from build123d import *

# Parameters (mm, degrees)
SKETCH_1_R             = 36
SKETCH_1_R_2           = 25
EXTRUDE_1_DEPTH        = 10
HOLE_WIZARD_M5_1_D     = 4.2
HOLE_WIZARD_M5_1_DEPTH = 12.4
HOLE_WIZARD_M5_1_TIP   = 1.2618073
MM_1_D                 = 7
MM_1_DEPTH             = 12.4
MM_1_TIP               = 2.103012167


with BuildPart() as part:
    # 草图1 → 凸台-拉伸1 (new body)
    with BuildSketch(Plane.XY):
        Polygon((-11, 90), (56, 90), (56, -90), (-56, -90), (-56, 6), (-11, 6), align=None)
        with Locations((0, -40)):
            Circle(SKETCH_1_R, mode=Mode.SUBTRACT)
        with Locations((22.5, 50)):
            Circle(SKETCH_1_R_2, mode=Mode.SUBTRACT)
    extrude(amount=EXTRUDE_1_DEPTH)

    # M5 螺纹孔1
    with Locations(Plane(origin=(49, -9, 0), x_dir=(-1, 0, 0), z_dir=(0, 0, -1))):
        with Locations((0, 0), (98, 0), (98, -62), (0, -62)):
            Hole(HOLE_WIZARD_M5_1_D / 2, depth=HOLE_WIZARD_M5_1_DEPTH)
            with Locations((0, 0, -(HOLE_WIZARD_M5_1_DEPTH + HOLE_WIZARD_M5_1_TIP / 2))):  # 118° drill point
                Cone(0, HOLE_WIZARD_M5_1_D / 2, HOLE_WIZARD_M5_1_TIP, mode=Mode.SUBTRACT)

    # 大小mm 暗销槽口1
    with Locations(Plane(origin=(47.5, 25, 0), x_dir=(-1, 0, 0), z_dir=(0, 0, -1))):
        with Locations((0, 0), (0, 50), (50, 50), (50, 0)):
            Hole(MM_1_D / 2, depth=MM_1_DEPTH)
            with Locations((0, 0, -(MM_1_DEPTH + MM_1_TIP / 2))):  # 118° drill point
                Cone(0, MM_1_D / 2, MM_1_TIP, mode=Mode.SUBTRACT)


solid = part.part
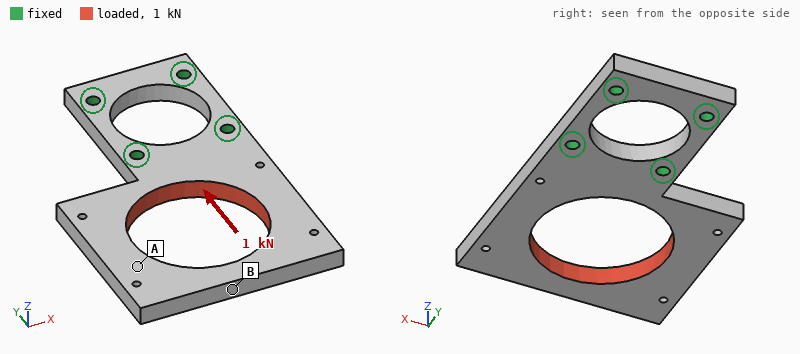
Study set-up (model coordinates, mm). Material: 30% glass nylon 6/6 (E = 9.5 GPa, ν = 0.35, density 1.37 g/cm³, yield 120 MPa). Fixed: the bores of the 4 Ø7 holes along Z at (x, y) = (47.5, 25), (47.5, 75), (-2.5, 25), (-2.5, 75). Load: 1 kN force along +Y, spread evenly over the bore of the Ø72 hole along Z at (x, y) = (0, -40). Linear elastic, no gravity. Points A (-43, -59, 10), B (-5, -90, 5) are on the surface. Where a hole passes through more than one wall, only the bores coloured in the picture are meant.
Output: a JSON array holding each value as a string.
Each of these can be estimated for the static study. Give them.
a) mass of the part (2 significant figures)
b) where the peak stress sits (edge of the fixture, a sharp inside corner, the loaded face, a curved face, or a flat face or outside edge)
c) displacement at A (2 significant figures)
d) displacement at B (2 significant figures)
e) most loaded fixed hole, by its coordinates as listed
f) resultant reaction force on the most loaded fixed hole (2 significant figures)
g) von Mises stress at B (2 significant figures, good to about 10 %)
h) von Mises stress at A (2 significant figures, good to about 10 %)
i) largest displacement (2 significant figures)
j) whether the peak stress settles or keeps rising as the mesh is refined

["140 g", "a sharp inside corner", "0.27 mm", "0.28 mm", "(-2.5, 25)", "920 N", "6.1 MPa", "2.1 MPa", "0.29 mm", "keeps rising"]
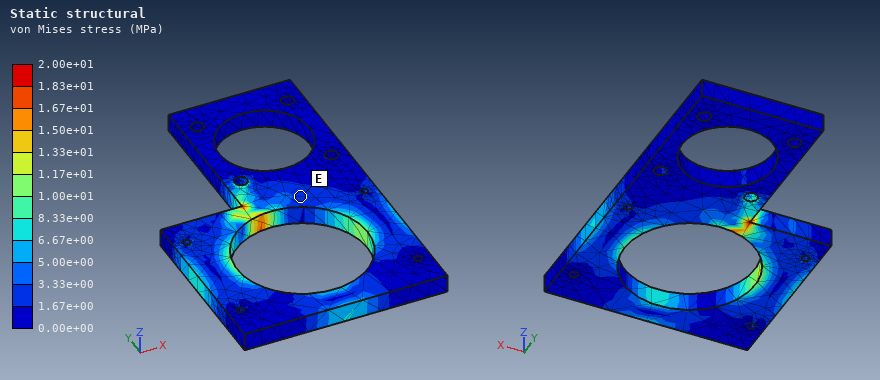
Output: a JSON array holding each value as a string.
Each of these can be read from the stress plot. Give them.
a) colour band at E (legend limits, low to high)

["1.67e+00 to 3.33e+00 MPa"]
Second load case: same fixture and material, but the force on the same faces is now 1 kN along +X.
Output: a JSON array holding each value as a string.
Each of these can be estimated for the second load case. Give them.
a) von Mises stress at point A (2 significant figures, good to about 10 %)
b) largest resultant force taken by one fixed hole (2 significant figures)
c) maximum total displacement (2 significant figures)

["2.1 MPa", "1.4 kN", "0.52 mm"]
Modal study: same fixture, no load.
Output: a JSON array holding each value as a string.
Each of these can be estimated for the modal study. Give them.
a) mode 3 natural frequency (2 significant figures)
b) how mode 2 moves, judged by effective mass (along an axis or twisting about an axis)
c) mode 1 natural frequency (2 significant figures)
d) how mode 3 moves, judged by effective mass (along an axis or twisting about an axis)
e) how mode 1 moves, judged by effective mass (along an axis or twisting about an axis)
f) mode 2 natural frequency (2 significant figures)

["730 Hz", "twisting about Y", "220 Hz", "along X", "along Z", "460 Hz"]
